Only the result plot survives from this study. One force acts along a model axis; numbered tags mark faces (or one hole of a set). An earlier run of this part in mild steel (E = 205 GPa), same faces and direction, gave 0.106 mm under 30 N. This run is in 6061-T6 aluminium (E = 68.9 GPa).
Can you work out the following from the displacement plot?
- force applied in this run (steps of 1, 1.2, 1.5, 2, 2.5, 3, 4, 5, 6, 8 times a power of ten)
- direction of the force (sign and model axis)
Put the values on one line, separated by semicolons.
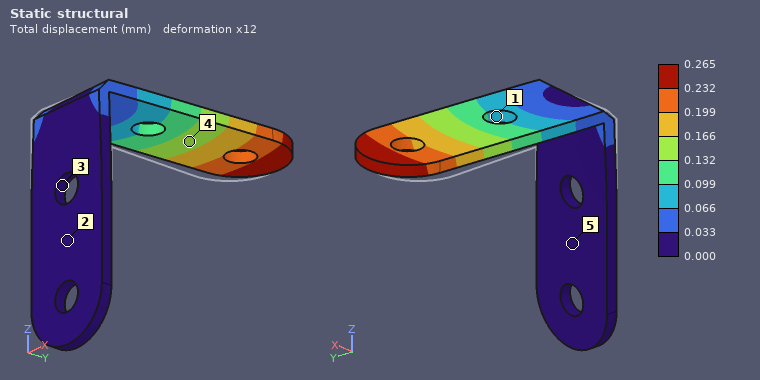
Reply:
25 N; +X
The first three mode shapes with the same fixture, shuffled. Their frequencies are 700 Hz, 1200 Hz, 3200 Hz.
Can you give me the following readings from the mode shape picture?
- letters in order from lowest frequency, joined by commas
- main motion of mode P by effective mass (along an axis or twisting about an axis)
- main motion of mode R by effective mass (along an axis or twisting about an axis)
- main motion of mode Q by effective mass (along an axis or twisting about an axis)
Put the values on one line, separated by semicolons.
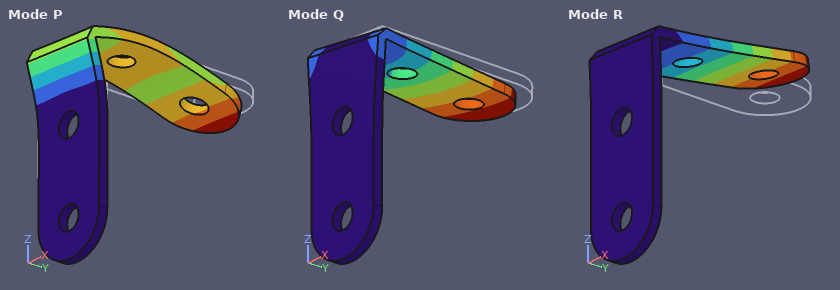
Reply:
R, Q, P; along Y; along Z; along X
